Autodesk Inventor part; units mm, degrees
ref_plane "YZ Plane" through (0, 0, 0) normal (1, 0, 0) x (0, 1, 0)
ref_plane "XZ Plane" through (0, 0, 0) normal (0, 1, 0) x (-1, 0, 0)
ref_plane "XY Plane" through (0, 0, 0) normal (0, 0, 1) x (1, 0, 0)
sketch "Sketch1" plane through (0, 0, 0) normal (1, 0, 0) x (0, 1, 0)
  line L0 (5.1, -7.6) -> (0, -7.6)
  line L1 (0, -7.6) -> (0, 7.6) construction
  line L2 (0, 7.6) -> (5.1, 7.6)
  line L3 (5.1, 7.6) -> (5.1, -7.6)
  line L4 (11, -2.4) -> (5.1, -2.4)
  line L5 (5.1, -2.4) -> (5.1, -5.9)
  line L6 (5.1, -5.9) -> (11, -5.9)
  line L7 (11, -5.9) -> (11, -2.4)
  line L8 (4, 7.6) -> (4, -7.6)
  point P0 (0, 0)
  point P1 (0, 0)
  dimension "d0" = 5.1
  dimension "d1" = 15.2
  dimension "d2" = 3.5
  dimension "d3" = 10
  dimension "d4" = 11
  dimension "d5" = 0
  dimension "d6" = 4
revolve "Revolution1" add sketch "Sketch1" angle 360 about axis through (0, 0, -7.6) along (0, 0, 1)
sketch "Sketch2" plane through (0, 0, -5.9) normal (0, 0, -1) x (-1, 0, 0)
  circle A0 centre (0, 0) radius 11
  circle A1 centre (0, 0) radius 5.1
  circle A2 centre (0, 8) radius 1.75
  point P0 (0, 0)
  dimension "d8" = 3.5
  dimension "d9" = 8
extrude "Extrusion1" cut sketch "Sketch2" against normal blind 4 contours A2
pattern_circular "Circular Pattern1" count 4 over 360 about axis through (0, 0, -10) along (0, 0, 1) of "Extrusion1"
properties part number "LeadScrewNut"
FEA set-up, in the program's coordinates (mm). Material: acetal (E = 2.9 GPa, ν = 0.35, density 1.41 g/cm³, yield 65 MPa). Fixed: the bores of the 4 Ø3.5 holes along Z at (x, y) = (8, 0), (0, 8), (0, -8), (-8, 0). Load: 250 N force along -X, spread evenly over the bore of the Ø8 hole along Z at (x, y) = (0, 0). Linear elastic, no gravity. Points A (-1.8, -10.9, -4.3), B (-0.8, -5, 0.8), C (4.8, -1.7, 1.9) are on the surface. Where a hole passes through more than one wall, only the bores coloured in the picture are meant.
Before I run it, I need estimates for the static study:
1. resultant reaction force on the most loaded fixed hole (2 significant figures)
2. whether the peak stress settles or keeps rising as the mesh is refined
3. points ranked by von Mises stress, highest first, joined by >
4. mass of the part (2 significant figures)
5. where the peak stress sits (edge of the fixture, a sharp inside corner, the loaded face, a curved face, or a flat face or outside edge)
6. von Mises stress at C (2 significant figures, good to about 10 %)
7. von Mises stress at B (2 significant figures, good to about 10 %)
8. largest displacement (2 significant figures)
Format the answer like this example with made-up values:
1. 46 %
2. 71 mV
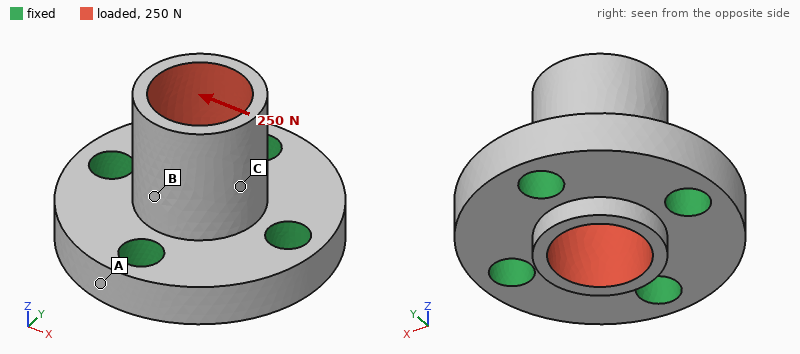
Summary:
1. 100 N
2. keeps rising
3. B > C > A
4. 2.0 g
5. a sharp inside corner
6. 4.8 MPa
7. 10 MPa
8. 0.10 mm
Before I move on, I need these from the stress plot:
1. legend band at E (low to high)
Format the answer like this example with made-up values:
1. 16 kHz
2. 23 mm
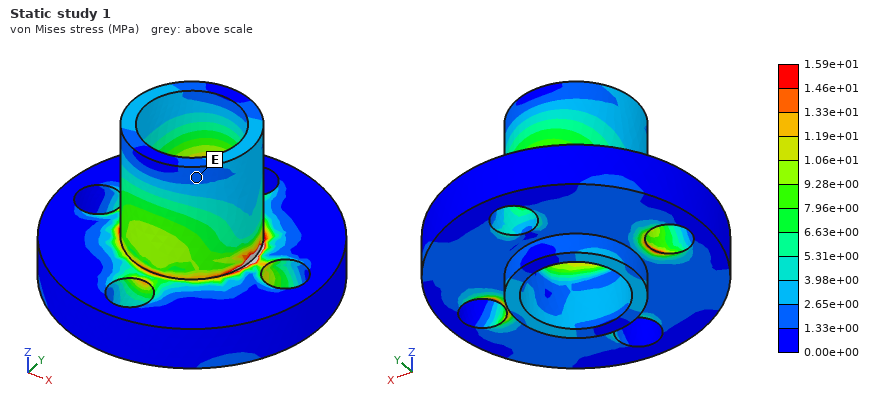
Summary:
1. 1.33e+00 to 2.65e+00 MPa
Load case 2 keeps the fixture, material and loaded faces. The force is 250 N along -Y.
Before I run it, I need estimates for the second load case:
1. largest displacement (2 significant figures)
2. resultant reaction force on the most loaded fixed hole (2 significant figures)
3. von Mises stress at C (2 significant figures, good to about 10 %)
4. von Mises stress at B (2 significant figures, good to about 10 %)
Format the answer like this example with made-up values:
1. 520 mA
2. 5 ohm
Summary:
1. 0.10 mm
2. 100 N
3. 8.8 MPa
4. 4.4 MPa
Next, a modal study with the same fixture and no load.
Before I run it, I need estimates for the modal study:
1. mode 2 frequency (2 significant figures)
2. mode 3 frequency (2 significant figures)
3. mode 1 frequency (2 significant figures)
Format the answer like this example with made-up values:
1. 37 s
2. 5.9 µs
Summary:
1. 11 kHz
2. 12 kHz
3. 11 kHz
